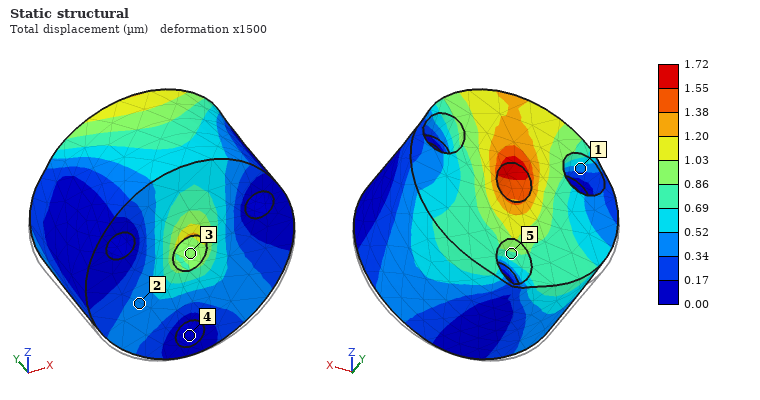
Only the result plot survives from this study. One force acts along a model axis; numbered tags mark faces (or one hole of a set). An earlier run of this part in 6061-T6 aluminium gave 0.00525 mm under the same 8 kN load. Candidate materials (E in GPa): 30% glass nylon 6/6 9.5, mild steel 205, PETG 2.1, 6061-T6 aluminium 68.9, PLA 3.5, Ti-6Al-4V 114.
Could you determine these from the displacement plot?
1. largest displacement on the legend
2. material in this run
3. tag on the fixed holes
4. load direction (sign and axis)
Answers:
1.72 µm
mild steel
4
+Z
